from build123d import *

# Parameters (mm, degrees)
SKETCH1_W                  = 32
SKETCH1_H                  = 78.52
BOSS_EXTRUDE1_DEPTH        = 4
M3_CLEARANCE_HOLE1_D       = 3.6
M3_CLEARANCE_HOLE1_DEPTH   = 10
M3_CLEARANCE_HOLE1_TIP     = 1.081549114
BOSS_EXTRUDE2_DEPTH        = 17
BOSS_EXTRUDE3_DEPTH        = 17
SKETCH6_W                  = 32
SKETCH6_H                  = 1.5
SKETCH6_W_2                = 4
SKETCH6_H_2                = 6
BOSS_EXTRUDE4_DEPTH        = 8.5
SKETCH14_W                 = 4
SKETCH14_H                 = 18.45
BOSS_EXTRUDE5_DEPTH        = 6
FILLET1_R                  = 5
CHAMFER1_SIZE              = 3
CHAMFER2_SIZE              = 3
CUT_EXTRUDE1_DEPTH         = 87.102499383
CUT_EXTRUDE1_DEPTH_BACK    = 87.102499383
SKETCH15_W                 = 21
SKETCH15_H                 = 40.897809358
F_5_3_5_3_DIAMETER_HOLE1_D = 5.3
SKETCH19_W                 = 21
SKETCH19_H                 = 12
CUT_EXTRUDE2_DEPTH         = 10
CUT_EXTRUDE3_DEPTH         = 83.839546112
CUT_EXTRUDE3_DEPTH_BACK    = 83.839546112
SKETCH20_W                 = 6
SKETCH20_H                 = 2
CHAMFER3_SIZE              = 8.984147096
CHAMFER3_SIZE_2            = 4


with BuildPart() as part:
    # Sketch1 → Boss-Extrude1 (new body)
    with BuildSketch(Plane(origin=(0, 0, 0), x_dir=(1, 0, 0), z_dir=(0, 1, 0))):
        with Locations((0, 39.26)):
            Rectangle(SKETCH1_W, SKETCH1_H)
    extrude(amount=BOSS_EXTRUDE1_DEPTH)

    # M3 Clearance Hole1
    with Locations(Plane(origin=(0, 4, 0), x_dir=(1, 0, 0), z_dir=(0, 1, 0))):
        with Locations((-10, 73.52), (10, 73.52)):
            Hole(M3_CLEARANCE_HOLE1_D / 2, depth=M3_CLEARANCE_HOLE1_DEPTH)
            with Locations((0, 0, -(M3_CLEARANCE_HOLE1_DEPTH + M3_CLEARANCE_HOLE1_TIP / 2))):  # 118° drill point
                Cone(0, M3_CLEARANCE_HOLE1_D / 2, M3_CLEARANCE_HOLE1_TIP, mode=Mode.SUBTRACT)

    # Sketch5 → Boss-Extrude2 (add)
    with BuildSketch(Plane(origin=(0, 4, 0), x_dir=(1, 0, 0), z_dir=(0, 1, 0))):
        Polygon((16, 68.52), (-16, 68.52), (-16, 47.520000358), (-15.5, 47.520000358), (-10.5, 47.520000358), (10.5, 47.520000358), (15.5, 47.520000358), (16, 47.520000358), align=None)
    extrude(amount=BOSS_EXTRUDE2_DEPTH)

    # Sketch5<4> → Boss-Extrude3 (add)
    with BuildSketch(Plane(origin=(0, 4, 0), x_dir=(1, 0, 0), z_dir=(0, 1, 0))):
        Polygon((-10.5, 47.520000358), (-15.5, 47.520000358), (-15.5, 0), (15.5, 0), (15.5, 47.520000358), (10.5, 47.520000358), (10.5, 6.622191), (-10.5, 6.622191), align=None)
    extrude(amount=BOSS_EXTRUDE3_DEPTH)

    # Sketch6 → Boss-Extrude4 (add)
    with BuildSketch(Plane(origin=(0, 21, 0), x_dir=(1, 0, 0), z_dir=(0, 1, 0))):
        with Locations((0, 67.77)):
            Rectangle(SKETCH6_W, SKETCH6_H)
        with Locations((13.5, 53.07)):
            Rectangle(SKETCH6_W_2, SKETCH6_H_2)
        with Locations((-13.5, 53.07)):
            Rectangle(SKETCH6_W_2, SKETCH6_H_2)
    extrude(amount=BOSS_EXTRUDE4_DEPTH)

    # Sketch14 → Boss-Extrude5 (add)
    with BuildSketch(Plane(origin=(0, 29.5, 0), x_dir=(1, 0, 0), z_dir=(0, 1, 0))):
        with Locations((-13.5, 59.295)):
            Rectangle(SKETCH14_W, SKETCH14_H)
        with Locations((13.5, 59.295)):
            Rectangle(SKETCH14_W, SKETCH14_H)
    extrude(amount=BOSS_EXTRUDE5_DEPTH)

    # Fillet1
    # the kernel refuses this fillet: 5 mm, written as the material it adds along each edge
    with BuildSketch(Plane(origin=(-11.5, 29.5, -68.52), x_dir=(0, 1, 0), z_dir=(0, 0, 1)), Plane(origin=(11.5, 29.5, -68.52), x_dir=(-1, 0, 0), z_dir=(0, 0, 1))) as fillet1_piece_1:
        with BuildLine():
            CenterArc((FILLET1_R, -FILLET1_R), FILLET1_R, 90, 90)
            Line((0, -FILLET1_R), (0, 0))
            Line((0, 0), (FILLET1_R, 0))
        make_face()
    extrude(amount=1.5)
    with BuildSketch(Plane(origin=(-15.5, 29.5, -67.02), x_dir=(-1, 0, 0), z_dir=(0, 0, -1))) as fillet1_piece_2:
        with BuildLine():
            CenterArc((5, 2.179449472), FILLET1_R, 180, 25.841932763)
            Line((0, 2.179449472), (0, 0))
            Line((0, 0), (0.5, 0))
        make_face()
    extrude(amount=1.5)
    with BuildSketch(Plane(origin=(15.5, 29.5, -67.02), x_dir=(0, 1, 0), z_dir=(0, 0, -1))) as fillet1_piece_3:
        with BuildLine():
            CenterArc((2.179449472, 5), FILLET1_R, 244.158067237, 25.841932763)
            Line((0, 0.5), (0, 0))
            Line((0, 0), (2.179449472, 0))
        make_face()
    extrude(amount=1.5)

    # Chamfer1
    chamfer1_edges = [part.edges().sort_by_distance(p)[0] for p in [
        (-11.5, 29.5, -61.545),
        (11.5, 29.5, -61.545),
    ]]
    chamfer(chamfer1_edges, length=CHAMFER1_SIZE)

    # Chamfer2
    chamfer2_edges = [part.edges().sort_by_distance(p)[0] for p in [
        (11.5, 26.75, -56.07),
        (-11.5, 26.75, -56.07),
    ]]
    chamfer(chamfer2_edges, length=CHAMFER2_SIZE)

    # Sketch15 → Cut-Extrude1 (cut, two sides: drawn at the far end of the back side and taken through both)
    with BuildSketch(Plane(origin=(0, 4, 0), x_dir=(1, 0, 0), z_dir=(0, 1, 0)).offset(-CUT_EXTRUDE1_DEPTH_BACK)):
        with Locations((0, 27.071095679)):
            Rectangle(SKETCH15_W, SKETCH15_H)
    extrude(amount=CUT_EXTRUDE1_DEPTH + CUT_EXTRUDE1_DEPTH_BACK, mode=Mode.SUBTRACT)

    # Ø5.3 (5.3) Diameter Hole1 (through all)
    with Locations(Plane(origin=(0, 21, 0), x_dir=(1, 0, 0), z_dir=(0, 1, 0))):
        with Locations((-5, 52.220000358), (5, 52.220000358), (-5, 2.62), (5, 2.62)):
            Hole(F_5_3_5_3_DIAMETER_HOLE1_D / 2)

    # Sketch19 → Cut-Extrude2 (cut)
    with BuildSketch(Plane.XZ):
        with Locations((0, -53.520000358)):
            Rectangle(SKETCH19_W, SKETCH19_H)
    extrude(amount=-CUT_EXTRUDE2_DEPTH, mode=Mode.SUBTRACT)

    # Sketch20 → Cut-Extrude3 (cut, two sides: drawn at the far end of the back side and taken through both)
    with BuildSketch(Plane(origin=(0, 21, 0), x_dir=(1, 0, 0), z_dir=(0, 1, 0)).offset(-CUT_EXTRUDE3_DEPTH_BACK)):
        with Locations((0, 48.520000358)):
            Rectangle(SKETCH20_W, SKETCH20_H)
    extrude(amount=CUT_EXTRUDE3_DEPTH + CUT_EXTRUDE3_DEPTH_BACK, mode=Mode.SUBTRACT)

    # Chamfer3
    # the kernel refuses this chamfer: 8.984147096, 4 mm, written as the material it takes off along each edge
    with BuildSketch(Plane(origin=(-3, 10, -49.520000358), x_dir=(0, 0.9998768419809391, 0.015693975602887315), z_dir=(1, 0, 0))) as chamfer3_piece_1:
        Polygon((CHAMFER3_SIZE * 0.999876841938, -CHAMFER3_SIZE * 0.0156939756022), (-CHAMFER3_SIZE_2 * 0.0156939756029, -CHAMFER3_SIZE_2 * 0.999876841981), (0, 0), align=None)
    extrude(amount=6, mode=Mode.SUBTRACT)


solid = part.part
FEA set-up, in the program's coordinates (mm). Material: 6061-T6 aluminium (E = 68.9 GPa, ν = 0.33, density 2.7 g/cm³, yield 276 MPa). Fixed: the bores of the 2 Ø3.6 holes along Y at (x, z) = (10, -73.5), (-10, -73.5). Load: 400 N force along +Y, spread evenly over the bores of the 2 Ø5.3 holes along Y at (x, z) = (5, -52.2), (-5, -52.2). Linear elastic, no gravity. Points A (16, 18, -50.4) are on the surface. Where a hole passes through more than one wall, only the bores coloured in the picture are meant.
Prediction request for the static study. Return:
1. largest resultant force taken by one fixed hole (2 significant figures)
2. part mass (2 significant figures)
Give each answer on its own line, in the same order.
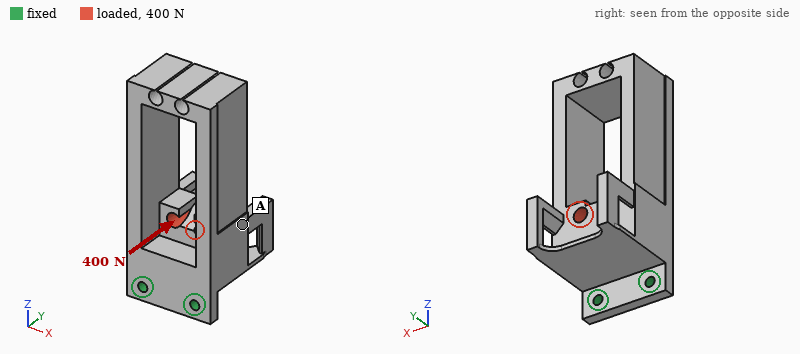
200 N
70 g
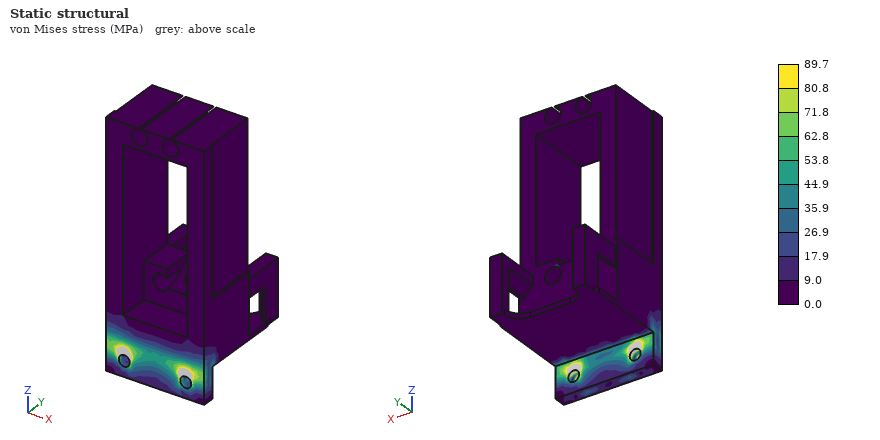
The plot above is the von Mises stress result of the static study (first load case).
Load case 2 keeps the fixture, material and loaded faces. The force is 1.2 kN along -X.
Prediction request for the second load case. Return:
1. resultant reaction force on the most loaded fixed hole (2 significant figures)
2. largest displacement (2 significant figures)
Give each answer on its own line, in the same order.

1.5 kN
50 µm
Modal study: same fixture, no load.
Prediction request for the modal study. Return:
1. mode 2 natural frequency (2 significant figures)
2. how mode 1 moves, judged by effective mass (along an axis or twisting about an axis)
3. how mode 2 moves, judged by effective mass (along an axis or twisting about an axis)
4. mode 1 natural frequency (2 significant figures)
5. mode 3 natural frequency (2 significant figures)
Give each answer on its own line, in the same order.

1400 Hz
along Y
along X
630 Hz
3300 Hz
